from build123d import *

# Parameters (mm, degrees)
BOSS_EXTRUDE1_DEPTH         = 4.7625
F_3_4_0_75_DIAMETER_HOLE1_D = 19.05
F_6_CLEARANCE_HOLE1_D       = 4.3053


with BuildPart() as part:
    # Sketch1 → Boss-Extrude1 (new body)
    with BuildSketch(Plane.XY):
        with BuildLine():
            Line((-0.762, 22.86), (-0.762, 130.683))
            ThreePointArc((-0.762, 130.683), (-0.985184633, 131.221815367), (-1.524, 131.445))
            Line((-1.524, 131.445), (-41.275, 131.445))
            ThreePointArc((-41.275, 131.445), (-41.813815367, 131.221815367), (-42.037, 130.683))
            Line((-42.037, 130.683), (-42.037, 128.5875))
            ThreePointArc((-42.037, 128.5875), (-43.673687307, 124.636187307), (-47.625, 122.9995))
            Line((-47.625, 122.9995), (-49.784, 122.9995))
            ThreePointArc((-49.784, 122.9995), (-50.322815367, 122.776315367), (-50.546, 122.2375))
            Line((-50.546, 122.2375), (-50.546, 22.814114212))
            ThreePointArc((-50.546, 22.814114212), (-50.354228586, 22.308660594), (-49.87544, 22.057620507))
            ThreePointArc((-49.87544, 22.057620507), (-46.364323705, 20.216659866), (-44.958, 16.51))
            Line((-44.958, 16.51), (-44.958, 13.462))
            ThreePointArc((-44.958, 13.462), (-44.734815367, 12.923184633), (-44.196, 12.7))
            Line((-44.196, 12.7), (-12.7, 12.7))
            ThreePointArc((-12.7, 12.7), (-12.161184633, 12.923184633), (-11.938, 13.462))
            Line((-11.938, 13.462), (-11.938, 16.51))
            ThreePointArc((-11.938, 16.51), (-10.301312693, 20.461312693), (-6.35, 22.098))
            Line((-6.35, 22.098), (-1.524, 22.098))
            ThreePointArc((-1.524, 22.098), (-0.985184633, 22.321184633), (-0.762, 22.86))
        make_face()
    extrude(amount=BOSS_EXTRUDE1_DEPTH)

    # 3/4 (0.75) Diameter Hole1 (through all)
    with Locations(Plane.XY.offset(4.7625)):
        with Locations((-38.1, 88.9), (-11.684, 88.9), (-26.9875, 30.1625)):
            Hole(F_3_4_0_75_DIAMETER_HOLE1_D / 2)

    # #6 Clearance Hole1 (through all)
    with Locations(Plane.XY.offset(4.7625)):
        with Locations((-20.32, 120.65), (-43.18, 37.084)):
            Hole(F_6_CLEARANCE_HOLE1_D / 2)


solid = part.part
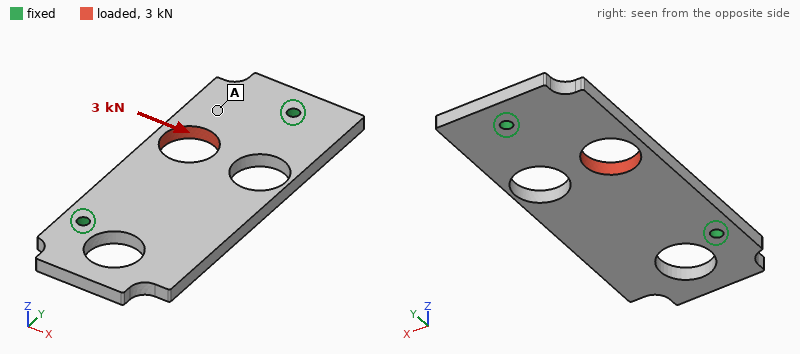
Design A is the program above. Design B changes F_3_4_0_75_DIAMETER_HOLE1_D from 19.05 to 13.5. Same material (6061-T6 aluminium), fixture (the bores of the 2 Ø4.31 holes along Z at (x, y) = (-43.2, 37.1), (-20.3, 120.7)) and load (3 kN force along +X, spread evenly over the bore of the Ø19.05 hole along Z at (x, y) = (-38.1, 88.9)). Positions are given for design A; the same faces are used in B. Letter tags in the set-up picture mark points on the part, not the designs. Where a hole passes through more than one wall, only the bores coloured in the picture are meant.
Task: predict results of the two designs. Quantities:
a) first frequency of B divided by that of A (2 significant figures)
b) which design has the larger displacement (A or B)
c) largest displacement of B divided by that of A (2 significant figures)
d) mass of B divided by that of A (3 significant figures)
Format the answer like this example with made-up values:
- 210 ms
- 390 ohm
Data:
- 1.1
- A
- 0.73
- 1.09
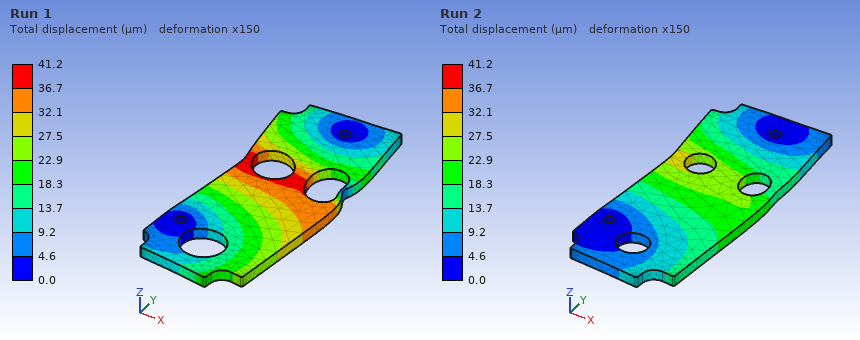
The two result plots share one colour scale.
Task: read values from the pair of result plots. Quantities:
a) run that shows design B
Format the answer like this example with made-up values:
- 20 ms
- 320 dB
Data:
- Run 2
